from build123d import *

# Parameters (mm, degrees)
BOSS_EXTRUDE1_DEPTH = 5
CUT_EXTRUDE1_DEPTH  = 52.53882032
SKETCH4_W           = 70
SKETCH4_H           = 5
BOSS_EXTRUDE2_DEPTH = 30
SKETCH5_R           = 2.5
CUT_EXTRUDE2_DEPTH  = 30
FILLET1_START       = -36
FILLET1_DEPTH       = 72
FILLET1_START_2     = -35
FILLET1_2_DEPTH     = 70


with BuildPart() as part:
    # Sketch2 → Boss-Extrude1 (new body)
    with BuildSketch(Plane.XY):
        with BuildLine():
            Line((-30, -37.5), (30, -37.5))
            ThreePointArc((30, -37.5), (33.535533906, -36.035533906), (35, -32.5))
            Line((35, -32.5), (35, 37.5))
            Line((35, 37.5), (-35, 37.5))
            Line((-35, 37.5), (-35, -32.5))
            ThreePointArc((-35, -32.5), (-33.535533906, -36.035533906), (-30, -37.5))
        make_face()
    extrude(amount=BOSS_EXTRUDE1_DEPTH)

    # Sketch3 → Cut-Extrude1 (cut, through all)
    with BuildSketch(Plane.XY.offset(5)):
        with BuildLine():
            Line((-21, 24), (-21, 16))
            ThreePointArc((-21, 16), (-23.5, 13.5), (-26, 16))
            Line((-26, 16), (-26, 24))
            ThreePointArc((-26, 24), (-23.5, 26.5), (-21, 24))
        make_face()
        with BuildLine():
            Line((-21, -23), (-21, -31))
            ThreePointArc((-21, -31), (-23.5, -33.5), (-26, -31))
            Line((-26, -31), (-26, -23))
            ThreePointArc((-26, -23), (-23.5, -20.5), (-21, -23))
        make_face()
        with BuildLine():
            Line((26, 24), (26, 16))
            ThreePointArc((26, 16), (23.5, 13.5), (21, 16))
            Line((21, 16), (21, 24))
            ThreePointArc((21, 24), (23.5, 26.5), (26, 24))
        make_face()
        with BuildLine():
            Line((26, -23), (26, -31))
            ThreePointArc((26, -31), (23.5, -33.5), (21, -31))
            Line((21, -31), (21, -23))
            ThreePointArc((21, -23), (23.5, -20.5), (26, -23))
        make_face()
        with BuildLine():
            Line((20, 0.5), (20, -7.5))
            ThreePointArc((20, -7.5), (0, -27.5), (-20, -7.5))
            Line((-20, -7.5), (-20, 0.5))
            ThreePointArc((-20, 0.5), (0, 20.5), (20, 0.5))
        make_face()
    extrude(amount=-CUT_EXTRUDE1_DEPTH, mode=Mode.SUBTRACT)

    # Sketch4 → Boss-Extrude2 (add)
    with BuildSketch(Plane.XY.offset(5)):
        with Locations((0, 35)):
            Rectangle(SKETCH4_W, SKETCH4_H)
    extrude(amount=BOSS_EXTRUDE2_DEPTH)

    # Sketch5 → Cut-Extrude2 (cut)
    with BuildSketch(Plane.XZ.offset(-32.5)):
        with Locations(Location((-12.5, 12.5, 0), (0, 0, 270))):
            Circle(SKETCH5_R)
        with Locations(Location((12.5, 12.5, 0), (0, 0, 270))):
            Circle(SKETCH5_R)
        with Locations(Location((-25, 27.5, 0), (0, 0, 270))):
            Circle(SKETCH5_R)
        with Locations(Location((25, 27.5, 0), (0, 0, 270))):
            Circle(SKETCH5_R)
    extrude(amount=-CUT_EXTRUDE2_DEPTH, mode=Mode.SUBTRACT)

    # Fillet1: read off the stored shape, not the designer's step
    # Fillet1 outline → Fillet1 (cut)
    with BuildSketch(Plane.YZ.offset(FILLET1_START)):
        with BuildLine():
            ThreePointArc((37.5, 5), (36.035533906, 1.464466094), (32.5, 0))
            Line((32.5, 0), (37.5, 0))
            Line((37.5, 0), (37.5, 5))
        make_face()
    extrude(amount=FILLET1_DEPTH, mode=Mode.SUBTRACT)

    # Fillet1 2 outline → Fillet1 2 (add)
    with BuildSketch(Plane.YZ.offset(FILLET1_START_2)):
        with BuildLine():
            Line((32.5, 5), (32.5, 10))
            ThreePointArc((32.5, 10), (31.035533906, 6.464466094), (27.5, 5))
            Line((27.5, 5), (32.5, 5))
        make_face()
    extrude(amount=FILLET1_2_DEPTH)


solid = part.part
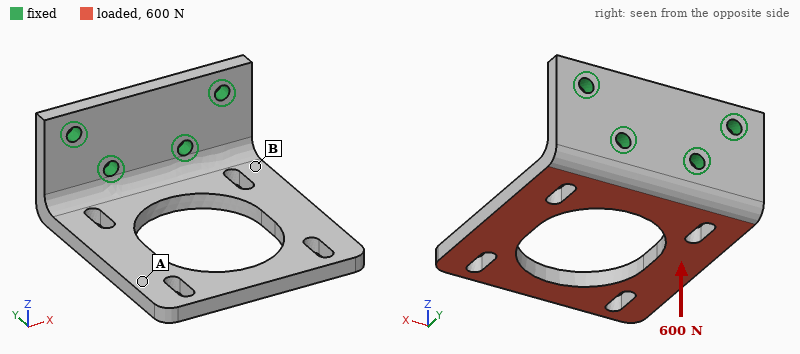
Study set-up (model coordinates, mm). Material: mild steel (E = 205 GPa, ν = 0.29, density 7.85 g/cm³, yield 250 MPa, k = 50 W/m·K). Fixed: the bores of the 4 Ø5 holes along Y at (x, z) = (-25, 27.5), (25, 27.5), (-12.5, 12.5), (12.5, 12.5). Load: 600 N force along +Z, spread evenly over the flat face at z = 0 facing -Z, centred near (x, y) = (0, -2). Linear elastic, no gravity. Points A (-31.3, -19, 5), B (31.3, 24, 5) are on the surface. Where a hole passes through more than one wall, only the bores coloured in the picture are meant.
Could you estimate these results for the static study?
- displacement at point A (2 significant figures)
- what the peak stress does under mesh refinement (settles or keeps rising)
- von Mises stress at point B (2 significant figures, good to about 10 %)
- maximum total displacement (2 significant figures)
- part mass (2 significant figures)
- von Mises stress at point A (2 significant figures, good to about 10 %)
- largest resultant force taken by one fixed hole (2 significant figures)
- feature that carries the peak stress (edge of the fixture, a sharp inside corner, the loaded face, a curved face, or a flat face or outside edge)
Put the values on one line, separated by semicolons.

0.25 mm; keeps rising; 93 MPa; 0.39 mm; 210 g; 16 MPa; 360 N; edge of the fixture
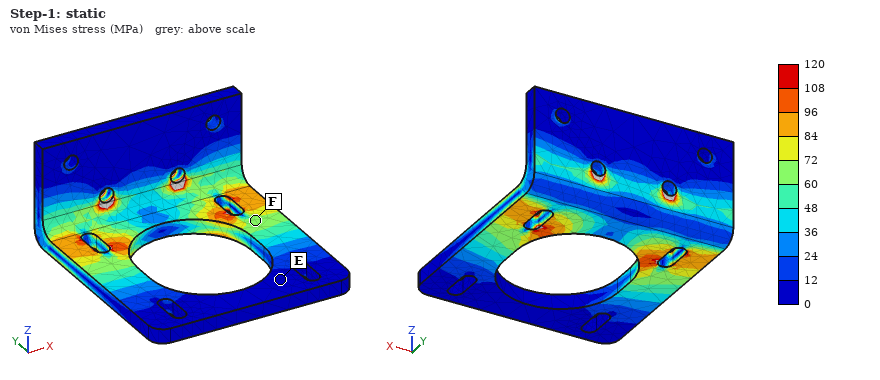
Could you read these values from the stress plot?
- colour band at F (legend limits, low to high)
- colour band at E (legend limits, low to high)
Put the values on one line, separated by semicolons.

60 to 72 MPa; 0 to 12 MPa
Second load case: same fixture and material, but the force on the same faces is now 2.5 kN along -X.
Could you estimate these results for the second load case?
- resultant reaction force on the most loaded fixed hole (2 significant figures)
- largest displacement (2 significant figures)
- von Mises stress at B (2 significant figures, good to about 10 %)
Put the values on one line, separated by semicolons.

2.8 kN; 0.11 mm; 63 MPa
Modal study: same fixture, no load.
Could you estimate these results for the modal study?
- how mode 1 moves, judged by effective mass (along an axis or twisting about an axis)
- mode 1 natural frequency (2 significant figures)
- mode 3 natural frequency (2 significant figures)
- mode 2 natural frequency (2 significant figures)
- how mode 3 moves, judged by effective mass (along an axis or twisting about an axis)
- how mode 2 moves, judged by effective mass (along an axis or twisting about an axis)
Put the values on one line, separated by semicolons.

along Z; 680 Hz; 2500 Hz; 1500 Hz; along X; twisting about Y
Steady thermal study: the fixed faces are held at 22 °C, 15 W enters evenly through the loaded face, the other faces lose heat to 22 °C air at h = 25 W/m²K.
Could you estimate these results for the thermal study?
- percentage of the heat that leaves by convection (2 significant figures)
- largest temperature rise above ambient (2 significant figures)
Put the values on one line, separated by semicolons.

30 %; 46 K
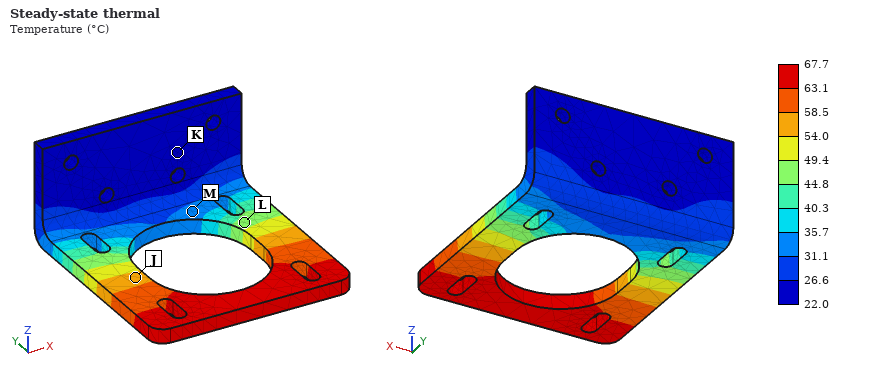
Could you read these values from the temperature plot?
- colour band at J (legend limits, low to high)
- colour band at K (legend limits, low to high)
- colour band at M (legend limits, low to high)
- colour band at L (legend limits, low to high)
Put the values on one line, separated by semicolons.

54.0 to 58.5 °C; 22.0 to 26.6 °C; 31.1 to 35.7 °C; 44.8 to 49.4 °C
